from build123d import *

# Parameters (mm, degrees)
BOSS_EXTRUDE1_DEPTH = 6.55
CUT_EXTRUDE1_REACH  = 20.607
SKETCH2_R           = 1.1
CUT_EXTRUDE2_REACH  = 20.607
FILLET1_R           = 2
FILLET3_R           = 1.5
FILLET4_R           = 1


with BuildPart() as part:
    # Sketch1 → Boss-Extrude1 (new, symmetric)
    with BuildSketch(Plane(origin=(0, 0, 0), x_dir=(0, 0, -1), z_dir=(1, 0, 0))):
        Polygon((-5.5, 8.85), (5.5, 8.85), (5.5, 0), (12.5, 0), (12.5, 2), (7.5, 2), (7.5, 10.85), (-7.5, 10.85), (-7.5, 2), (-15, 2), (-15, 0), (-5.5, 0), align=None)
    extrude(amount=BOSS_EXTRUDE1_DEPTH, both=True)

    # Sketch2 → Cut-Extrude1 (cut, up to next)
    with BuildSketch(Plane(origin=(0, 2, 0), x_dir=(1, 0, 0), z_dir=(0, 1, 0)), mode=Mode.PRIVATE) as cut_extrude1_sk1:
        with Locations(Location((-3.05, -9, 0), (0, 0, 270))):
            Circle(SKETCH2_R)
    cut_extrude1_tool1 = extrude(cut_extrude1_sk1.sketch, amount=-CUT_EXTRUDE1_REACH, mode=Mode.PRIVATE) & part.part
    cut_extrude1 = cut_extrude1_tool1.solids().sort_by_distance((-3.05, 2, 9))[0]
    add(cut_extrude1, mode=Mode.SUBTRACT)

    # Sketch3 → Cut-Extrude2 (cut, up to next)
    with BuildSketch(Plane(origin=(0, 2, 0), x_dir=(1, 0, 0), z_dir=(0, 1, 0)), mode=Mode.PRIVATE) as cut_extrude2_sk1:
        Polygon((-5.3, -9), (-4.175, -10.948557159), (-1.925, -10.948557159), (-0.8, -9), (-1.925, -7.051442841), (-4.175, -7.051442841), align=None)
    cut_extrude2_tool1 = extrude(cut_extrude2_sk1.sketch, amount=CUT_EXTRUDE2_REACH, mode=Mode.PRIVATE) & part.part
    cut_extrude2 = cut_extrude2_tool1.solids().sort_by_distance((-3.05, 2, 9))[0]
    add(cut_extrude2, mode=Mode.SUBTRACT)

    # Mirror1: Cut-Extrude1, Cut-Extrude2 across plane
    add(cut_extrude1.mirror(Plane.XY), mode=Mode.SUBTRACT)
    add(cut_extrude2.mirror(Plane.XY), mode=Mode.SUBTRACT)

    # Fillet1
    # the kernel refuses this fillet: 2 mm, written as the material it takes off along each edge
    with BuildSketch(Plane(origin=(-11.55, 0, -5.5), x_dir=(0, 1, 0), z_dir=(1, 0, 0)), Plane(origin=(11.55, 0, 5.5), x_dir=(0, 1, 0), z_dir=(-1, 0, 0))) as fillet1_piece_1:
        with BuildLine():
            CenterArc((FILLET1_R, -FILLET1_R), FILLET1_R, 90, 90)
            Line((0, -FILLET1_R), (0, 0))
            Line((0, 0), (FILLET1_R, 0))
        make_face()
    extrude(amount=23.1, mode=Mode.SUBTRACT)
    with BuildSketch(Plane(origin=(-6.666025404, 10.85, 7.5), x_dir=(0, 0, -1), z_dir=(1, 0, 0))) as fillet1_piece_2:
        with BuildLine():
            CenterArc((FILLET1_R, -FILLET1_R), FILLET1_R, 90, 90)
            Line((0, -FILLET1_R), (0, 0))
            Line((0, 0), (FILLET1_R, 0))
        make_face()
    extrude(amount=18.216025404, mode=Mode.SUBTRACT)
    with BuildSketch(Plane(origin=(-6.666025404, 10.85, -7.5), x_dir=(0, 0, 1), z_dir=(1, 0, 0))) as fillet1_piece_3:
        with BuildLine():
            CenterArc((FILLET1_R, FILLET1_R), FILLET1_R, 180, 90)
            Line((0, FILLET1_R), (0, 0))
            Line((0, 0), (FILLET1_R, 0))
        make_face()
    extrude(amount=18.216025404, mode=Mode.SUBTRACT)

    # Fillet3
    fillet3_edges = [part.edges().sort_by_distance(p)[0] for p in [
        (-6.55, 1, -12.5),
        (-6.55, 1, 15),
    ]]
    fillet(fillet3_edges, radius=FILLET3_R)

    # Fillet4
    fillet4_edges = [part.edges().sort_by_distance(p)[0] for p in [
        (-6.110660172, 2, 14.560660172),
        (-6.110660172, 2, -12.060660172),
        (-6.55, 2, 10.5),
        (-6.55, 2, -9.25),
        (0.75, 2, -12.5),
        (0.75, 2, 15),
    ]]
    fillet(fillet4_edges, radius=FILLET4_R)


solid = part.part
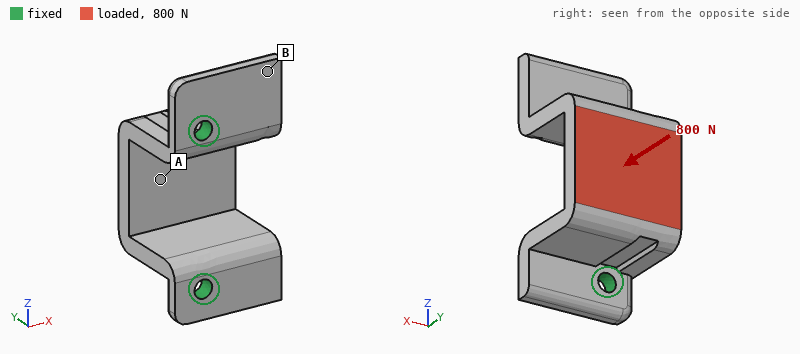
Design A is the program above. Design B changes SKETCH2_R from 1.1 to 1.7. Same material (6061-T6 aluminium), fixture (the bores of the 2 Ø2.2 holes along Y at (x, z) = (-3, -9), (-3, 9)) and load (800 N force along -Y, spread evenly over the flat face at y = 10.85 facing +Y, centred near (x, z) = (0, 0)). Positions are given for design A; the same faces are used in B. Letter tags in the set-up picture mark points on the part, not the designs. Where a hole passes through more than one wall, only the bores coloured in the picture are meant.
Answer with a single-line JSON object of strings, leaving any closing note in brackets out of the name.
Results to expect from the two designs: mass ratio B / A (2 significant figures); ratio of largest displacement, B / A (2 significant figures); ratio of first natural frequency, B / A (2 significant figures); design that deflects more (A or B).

{"mass ratio B / A": "0.98", "ratio of largest displacement, B / A": "0.68", "ratio of first natural frequency, B / A": "1.3", "design that deflects more": "A"}
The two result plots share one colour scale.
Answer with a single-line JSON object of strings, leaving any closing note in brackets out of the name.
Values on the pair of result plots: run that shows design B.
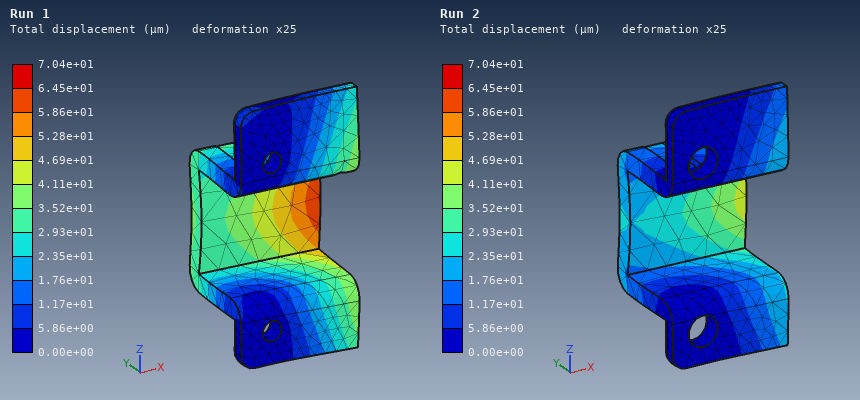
{"run that shows design B": "Run 2"}
